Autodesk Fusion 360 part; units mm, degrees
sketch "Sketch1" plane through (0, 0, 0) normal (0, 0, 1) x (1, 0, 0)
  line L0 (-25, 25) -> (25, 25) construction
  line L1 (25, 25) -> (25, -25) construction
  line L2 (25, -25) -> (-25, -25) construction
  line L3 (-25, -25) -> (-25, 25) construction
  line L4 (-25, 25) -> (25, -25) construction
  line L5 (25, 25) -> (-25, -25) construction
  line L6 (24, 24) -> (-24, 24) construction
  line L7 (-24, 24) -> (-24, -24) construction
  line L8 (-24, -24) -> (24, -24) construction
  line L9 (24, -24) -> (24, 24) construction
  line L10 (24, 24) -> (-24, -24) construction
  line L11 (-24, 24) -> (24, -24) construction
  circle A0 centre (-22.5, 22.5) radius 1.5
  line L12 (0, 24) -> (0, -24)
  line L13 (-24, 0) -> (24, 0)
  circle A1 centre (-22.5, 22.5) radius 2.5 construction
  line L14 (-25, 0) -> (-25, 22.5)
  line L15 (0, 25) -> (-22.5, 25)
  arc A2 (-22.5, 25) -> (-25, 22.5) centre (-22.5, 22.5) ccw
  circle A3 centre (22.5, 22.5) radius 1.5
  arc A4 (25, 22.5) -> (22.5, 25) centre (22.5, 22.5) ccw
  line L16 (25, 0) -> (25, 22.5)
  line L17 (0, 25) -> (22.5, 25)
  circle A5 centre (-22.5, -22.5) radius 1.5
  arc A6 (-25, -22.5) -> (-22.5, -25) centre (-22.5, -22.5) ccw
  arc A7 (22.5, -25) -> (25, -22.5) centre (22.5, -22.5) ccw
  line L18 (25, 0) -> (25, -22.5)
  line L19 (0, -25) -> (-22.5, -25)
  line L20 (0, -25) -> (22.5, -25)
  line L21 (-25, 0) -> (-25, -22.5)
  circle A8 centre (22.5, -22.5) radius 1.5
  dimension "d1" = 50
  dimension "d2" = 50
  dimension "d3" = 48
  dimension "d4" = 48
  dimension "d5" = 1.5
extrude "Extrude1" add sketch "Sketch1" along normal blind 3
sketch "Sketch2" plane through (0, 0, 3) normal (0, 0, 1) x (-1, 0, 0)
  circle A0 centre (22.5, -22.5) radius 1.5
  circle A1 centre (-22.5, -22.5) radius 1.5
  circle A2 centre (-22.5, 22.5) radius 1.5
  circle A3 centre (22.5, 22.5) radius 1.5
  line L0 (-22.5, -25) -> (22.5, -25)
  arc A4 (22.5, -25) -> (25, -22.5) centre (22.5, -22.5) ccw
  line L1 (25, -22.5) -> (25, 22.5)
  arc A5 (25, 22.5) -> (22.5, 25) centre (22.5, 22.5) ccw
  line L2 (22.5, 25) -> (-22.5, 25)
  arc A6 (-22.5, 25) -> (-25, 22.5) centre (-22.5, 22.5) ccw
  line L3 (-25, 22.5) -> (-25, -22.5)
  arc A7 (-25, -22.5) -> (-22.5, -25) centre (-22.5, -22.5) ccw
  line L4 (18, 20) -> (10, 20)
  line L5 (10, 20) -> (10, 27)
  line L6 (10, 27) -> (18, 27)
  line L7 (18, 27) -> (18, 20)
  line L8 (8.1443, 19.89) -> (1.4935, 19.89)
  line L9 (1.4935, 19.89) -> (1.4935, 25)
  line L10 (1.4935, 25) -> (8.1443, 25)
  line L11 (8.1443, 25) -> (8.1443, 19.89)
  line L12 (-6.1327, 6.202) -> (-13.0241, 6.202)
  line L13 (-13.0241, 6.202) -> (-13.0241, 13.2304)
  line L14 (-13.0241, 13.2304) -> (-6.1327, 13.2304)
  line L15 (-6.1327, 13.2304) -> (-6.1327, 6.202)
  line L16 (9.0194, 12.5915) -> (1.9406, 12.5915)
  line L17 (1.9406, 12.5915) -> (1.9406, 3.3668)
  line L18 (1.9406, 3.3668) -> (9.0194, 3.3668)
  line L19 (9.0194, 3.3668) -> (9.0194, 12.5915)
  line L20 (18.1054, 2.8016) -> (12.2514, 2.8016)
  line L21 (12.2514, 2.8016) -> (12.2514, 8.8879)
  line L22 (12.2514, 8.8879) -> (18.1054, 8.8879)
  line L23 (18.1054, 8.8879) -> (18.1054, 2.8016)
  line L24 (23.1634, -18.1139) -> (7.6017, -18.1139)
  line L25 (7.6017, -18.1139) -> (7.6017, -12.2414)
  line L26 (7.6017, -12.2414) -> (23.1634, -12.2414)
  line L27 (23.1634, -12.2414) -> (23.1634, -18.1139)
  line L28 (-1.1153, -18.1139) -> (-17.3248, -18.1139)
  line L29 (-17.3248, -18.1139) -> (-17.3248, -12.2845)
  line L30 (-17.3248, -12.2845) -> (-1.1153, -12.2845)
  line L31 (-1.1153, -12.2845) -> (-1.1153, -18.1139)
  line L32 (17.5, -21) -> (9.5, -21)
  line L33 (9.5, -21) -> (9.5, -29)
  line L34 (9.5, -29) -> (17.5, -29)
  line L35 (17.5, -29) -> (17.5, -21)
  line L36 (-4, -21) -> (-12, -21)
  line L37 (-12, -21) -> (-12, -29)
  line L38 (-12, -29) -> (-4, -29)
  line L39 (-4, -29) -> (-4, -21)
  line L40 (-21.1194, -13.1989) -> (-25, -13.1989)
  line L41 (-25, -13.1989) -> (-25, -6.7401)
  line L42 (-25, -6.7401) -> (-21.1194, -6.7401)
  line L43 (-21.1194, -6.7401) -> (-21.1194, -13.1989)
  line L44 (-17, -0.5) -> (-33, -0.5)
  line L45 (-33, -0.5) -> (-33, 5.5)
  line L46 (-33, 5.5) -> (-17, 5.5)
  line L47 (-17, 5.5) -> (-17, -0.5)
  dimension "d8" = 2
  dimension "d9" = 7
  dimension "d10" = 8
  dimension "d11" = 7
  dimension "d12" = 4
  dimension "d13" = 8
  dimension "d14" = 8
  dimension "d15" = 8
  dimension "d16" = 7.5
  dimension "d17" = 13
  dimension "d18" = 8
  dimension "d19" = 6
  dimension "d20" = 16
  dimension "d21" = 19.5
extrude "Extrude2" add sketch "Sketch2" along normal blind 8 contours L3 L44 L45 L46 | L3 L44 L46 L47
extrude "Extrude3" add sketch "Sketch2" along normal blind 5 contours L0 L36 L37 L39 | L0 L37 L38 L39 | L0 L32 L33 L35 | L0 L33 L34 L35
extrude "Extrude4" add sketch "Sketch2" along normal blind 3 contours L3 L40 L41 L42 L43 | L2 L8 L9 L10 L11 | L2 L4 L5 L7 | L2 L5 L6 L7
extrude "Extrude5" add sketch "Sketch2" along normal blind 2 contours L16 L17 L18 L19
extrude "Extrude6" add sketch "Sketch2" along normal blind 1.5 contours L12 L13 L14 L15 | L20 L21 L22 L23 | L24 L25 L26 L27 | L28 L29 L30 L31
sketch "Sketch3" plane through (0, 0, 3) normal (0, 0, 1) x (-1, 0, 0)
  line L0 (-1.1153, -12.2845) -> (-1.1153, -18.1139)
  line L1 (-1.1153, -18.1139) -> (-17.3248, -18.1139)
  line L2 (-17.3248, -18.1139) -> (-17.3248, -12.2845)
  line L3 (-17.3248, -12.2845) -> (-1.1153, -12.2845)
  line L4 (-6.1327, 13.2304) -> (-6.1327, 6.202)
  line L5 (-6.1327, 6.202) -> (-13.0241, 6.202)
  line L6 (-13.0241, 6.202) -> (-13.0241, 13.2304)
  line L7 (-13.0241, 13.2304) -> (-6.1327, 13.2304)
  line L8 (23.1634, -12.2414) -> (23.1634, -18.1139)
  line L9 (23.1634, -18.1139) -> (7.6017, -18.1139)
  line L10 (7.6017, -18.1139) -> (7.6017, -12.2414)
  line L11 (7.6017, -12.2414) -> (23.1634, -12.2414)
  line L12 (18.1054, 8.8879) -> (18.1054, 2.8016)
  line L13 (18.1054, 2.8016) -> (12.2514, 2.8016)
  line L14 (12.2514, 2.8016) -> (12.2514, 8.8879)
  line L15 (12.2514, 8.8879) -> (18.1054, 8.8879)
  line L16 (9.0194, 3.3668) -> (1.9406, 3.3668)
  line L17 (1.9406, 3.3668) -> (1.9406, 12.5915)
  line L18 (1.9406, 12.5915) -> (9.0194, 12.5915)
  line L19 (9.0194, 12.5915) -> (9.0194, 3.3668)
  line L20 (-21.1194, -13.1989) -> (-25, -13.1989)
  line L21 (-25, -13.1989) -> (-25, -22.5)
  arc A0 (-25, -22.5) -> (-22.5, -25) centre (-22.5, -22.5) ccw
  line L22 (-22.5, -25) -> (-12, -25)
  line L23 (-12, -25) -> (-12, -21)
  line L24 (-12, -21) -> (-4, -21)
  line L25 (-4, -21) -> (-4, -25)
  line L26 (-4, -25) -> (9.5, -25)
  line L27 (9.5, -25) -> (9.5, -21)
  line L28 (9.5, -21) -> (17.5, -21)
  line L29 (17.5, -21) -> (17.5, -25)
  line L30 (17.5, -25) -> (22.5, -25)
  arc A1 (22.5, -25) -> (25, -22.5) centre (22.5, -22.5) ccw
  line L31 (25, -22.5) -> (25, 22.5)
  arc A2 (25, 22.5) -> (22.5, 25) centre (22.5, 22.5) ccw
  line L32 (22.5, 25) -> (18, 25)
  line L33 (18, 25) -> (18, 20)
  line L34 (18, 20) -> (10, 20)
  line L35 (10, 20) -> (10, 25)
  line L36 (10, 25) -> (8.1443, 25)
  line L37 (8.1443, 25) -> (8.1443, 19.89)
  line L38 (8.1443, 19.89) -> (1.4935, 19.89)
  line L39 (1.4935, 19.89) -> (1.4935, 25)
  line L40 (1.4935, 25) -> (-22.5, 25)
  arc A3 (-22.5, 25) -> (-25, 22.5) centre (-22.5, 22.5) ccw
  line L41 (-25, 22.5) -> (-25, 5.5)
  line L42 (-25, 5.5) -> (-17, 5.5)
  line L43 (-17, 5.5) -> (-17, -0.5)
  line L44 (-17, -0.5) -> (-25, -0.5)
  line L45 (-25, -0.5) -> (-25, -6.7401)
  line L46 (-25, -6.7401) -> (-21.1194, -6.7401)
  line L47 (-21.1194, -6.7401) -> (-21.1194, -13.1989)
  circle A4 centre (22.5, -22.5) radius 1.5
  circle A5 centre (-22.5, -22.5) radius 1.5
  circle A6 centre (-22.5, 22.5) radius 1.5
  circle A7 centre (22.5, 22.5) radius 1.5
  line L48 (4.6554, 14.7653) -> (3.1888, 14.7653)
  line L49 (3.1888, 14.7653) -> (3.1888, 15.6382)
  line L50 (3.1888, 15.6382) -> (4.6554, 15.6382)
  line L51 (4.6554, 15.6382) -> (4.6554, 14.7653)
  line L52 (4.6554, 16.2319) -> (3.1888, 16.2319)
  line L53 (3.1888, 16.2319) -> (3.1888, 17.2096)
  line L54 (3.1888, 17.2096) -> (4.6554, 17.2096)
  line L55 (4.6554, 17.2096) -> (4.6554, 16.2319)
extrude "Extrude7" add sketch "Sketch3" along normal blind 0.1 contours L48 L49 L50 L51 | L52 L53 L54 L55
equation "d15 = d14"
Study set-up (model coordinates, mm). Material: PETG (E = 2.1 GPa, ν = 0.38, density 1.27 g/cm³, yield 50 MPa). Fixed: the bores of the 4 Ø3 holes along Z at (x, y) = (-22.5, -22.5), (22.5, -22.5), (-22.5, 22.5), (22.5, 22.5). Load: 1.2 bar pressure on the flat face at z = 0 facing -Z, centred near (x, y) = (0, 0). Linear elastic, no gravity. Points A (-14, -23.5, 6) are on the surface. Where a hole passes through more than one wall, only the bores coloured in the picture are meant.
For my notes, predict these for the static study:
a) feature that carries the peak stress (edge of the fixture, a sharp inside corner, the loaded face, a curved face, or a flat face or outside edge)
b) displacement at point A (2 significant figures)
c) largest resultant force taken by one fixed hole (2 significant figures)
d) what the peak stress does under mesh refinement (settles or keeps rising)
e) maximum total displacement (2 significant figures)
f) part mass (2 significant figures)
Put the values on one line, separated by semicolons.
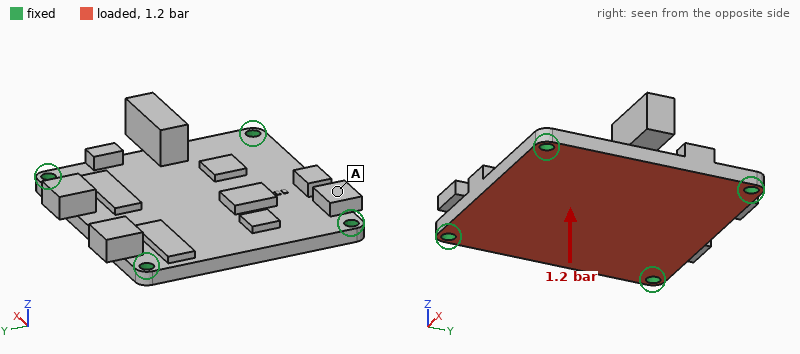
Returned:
edge of the fixture; 0.19 mm; 75 N; keeps rising; 0.69 mm; 12 g
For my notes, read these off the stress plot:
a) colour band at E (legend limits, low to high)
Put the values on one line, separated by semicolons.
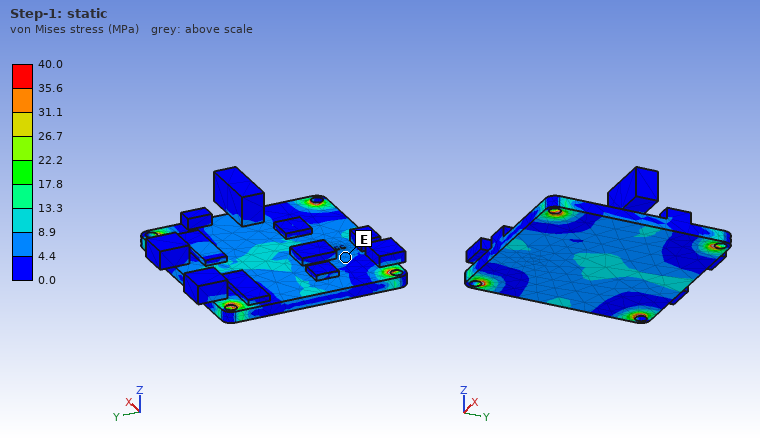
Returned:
4.4 to 8.9 MPa
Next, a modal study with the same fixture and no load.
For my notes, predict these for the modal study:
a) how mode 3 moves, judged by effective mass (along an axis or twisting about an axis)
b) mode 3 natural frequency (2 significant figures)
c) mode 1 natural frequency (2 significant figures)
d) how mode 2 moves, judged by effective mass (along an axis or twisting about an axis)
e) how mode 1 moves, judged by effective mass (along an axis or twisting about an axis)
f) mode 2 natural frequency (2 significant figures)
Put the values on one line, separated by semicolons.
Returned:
twisting about X; 1900 Hz; 1200 Hz; twisting about Y; along Z; 1400 Hz
